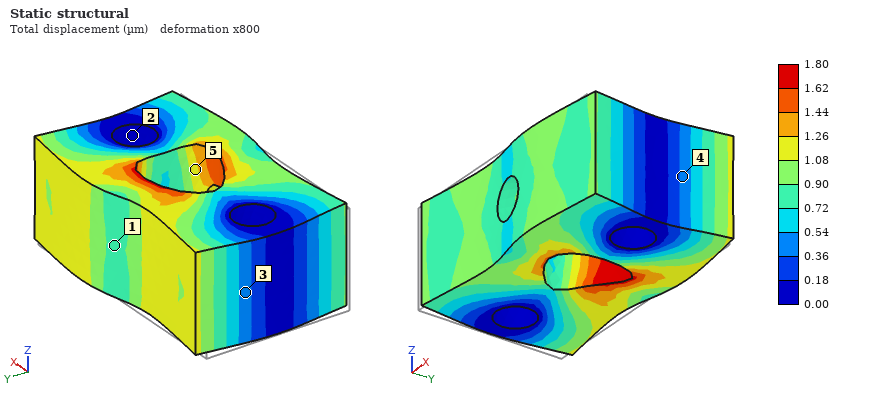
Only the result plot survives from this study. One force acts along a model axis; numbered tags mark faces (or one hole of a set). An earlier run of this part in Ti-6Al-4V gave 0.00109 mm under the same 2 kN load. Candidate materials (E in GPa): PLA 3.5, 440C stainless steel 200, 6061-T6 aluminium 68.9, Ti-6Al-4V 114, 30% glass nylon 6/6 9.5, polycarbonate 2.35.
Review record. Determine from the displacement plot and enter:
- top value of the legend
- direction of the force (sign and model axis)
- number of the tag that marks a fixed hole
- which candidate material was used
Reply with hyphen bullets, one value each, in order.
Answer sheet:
- 1.80 µm
- +X
- 2
- 6061-T6 aluminium
